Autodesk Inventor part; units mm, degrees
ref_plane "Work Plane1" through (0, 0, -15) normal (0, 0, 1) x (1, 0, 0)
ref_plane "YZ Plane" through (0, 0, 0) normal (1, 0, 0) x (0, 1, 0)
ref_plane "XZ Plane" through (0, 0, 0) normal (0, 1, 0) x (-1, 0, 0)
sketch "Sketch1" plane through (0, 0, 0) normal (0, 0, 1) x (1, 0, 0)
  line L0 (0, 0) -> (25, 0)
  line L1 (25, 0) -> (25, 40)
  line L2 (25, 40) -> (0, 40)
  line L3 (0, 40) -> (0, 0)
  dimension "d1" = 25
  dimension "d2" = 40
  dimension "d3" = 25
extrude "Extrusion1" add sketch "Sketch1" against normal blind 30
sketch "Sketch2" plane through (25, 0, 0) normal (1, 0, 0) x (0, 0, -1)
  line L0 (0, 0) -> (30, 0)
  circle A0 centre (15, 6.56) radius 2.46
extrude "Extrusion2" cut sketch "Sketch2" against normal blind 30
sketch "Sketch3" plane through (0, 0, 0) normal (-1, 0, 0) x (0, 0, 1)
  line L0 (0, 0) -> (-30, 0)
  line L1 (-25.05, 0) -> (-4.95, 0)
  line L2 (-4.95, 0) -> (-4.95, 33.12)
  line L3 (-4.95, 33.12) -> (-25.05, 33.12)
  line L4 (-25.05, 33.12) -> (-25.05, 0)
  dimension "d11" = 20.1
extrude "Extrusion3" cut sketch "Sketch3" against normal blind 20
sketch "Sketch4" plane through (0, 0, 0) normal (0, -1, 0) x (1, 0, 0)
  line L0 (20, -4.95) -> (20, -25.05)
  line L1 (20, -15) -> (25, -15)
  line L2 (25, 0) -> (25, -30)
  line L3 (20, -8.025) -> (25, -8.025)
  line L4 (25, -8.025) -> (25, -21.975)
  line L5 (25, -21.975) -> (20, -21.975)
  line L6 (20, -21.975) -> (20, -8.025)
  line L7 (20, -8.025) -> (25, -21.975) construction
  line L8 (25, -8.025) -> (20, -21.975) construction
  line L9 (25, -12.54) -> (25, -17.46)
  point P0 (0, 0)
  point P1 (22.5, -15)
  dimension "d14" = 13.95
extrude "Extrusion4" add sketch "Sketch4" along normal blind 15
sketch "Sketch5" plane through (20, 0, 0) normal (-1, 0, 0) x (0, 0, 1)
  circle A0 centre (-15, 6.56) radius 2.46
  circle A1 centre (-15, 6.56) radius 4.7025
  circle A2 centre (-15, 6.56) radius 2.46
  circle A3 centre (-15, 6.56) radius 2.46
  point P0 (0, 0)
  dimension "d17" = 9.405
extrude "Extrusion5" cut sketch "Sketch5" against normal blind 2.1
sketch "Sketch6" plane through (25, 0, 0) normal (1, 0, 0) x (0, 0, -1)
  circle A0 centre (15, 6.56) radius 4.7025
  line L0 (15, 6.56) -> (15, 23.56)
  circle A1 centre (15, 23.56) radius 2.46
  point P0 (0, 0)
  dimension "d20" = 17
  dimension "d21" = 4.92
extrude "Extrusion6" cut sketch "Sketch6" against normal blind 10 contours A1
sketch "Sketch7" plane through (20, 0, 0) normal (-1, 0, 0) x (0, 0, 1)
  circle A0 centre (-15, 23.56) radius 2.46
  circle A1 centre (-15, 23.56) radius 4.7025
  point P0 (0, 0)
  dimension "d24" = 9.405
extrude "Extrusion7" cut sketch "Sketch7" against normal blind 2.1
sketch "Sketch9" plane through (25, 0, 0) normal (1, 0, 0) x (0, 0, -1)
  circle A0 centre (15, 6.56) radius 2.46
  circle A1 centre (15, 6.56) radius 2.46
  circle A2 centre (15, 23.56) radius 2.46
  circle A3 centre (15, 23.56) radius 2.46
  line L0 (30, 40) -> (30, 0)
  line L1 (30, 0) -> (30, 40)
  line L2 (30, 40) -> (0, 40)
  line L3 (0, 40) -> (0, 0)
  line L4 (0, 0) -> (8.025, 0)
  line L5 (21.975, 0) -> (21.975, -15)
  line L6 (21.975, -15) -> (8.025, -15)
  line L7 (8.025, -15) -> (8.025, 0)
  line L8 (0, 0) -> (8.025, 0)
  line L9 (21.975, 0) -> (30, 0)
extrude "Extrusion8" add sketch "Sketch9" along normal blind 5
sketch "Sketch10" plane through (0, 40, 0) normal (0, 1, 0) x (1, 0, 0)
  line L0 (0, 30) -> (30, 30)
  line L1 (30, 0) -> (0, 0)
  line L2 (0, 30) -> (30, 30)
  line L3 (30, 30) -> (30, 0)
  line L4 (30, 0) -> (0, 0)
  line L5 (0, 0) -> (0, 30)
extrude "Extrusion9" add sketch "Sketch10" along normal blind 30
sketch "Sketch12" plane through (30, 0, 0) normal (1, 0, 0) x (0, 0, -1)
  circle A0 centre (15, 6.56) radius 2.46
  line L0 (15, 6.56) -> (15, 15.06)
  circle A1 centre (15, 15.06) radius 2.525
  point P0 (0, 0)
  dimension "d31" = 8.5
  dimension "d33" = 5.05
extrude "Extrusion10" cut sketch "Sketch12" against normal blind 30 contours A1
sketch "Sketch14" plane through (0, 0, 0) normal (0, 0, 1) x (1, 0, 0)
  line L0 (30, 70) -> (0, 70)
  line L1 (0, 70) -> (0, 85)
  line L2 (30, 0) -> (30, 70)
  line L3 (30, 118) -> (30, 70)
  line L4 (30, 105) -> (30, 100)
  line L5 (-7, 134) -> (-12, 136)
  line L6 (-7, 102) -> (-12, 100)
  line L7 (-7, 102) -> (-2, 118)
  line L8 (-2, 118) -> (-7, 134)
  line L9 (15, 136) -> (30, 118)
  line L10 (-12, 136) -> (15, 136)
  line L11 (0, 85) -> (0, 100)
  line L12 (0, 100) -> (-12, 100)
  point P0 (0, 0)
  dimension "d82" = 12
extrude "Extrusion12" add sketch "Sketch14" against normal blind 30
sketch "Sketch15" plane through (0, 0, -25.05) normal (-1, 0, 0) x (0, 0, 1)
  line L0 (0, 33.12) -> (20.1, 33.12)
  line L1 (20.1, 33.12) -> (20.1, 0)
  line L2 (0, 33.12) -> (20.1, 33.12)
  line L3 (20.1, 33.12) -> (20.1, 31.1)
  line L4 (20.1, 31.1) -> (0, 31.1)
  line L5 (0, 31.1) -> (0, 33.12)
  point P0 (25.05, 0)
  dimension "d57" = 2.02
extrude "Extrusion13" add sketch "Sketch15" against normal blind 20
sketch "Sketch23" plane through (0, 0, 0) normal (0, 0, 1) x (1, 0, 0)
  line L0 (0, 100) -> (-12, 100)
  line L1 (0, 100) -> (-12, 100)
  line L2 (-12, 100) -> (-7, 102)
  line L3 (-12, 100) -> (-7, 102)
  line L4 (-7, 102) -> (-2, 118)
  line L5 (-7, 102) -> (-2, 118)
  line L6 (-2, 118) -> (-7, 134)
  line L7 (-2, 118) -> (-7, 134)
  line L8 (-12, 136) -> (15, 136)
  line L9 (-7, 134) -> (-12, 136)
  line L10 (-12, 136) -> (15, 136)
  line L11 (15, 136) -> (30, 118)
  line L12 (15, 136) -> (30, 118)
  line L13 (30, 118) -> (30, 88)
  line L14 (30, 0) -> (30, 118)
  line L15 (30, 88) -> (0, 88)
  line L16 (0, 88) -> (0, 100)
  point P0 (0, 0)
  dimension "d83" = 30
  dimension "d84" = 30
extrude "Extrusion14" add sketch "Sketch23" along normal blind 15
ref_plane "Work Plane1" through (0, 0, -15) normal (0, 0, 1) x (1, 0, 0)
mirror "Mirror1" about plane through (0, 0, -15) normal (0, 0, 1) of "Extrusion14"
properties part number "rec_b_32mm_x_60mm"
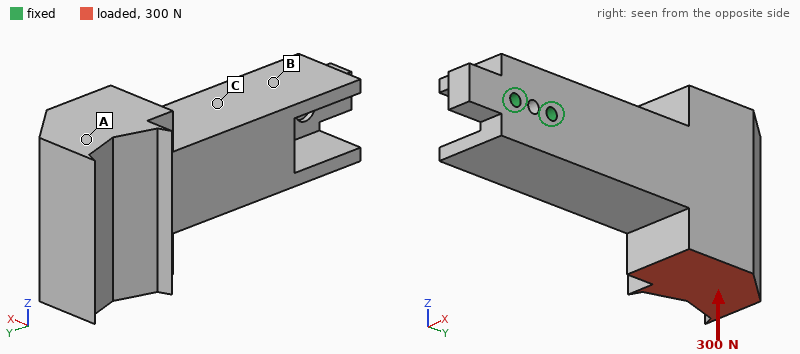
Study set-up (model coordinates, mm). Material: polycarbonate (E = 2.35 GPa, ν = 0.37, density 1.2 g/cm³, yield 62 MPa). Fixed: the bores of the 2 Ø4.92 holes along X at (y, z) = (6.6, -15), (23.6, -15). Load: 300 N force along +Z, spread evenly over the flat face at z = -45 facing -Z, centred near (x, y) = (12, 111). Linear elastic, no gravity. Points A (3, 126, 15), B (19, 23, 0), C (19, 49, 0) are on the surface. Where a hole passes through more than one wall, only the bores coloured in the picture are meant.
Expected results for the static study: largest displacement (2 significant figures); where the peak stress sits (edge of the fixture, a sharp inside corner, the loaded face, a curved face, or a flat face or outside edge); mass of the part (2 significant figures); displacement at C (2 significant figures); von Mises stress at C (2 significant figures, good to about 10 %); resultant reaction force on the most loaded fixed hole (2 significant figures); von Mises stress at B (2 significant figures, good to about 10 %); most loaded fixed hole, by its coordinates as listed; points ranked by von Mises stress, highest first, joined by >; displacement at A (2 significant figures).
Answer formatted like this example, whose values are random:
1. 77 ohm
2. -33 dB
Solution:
1. 2.0 mm
2. edge of the fixture
3. 190 g
4. 0.40 mm
5. 4.6 MPa
6. 1.4 kN
7. 9.9 MPa
8. (23.6, -15)
9. B > C > A
10. 1.8 mm
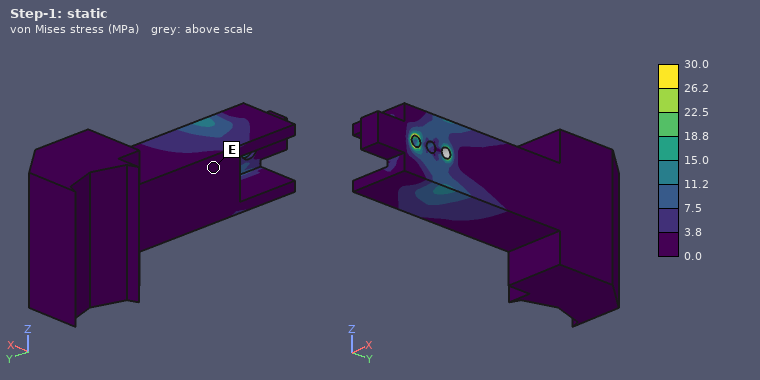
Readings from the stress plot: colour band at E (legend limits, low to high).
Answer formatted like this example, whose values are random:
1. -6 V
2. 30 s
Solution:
1. 0.0 to 3.8 MPa
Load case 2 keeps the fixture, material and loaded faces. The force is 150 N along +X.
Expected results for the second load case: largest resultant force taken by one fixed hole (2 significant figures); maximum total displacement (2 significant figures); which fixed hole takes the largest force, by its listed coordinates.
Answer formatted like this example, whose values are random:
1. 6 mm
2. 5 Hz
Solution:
1. 670 N
2. 1.6 mm
3. (23.6, -15)
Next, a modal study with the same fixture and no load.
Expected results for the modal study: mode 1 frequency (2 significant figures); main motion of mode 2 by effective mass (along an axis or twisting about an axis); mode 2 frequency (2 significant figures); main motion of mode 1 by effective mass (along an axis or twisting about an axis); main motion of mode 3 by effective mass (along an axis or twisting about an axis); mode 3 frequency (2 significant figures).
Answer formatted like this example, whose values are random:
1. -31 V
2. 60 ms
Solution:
1. 180 Hz
2. along Z
3. 210 Hz
4. along X
5. twisting about Y
6. 500 Hz
